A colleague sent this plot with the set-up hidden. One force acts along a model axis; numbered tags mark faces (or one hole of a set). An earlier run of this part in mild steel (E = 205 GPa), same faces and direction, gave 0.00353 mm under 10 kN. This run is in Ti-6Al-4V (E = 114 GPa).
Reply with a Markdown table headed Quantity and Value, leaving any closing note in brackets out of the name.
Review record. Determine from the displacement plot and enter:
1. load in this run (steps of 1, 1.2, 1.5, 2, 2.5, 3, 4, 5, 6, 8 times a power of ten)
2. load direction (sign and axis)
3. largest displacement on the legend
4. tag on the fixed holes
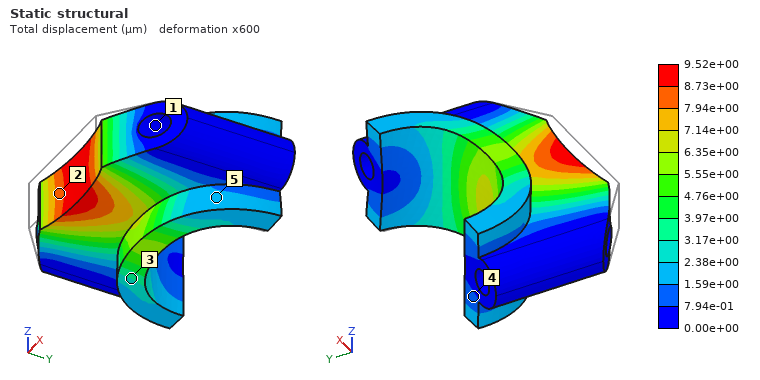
| Quantity | Value |
|---|---|
| load in this run | 15 kN |
| load direction | +Y |
| largest displacement on the legend | 9.52e+00 µm |
| tag on the fixed holes | 1 |
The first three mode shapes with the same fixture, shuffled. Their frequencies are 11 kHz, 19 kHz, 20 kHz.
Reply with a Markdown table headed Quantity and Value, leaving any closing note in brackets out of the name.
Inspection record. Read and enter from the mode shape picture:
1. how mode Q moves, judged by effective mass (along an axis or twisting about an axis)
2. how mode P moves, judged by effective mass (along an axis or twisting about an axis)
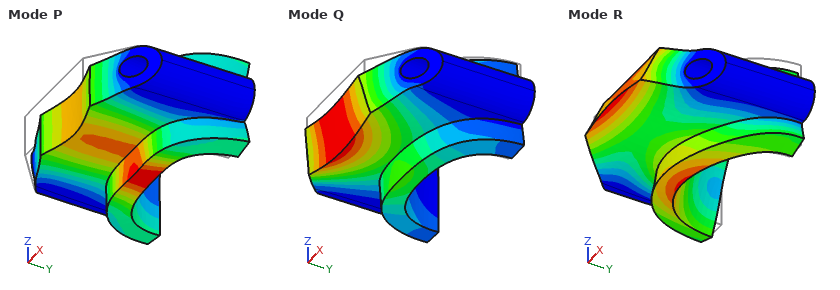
| Quantity | Value |
|---|---|
| how mode Q moves, judged by effective mass | along Z |
| how mode P moves, judged by effective mass | along Y |
